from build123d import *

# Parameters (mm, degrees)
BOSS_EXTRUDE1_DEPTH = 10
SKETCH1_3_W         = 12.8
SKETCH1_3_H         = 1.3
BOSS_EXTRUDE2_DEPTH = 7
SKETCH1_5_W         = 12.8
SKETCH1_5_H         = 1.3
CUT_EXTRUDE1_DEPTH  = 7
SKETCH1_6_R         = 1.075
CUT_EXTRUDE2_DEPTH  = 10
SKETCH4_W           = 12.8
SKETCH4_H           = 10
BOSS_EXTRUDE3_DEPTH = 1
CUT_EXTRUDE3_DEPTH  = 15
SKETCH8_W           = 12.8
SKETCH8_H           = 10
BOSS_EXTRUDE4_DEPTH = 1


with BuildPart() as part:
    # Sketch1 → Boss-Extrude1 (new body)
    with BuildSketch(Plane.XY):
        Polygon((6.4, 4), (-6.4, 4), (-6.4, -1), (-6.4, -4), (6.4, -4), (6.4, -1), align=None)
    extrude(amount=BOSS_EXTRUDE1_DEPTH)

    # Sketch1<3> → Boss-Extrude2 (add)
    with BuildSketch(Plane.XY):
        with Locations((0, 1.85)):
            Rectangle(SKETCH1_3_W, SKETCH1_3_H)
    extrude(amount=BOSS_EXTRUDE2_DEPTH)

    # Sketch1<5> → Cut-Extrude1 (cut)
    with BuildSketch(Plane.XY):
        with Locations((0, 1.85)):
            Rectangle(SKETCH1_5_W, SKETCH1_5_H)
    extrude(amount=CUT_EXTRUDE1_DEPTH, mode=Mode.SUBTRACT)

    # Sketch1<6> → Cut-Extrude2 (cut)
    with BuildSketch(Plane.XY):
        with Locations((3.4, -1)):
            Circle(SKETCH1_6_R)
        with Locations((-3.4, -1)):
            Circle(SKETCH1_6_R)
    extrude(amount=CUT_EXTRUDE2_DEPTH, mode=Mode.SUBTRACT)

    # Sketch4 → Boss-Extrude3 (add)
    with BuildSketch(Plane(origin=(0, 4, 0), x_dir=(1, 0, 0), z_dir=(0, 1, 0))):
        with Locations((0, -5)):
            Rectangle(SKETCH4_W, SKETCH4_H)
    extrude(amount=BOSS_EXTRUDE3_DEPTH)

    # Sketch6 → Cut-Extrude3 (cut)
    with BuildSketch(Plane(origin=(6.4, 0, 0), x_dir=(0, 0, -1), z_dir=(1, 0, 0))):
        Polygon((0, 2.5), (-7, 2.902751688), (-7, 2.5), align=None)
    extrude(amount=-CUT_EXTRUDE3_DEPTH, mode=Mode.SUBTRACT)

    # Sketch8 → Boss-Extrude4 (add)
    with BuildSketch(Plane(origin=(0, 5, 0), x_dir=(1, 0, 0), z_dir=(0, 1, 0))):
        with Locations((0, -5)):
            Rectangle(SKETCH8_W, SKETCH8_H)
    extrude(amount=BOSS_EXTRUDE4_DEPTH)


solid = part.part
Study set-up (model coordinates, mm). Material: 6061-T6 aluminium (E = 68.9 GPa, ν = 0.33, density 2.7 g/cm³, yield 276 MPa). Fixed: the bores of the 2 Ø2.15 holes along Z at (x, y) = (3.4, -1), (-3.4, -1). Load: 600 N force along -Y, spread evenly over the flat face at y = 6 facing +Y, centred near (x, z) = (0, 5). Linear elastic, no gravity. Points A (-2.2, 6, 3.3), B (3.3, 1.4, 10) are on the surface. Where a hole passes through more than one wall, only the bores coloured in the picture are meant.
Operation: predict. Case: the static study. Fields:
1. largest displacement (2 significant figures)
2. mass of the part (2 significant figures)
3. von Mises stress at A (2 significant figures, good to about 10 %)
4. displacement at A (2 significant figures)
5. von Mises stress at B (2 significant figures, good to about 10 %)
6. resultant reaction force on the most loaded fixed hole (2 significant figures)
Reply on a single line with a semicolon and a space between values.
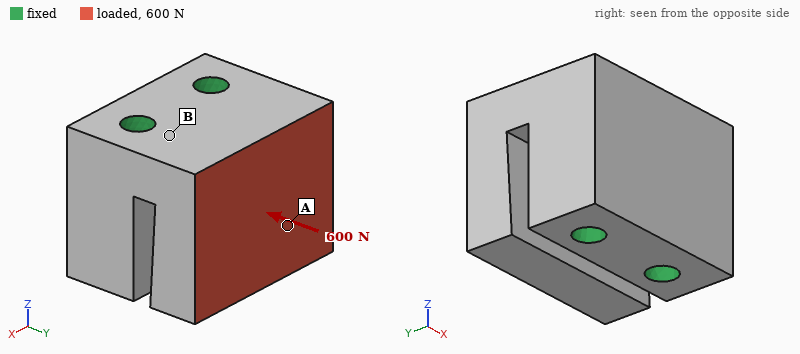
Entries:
50 µm; 2.9 g; 16 MPa; 33 µm; 86 MPa; 310 N
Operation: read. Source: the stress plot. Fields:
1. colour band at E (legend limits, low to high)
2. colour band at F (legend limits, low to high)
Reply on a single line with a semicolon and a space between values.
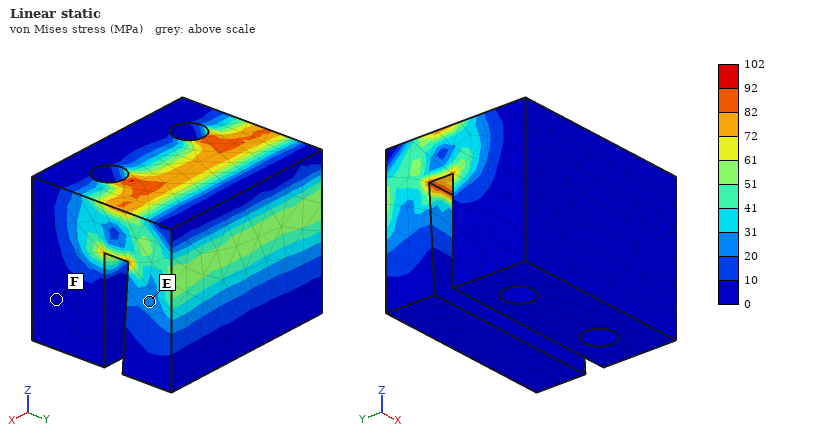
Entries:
20 to 31 MPa; 0 to 10 MPa
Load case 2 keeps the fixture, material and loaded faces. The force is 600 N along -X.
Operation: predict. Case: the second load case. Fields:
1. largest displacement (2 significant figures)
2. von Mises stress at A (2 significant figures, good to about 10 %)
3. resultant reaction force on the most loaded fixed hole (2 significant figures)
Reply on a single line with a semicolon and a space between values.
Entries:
18 µm; 20 MPa; 580 N
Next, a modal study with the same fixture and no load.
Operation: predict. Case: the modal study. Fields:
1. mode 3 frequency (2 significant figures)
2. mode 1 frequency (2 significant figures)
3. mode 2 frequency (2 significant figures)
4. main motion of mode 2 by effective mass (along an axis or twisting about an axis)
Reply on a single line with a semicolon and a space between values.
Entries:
46 kHz; 18 kHz; 30 kHz; along X
